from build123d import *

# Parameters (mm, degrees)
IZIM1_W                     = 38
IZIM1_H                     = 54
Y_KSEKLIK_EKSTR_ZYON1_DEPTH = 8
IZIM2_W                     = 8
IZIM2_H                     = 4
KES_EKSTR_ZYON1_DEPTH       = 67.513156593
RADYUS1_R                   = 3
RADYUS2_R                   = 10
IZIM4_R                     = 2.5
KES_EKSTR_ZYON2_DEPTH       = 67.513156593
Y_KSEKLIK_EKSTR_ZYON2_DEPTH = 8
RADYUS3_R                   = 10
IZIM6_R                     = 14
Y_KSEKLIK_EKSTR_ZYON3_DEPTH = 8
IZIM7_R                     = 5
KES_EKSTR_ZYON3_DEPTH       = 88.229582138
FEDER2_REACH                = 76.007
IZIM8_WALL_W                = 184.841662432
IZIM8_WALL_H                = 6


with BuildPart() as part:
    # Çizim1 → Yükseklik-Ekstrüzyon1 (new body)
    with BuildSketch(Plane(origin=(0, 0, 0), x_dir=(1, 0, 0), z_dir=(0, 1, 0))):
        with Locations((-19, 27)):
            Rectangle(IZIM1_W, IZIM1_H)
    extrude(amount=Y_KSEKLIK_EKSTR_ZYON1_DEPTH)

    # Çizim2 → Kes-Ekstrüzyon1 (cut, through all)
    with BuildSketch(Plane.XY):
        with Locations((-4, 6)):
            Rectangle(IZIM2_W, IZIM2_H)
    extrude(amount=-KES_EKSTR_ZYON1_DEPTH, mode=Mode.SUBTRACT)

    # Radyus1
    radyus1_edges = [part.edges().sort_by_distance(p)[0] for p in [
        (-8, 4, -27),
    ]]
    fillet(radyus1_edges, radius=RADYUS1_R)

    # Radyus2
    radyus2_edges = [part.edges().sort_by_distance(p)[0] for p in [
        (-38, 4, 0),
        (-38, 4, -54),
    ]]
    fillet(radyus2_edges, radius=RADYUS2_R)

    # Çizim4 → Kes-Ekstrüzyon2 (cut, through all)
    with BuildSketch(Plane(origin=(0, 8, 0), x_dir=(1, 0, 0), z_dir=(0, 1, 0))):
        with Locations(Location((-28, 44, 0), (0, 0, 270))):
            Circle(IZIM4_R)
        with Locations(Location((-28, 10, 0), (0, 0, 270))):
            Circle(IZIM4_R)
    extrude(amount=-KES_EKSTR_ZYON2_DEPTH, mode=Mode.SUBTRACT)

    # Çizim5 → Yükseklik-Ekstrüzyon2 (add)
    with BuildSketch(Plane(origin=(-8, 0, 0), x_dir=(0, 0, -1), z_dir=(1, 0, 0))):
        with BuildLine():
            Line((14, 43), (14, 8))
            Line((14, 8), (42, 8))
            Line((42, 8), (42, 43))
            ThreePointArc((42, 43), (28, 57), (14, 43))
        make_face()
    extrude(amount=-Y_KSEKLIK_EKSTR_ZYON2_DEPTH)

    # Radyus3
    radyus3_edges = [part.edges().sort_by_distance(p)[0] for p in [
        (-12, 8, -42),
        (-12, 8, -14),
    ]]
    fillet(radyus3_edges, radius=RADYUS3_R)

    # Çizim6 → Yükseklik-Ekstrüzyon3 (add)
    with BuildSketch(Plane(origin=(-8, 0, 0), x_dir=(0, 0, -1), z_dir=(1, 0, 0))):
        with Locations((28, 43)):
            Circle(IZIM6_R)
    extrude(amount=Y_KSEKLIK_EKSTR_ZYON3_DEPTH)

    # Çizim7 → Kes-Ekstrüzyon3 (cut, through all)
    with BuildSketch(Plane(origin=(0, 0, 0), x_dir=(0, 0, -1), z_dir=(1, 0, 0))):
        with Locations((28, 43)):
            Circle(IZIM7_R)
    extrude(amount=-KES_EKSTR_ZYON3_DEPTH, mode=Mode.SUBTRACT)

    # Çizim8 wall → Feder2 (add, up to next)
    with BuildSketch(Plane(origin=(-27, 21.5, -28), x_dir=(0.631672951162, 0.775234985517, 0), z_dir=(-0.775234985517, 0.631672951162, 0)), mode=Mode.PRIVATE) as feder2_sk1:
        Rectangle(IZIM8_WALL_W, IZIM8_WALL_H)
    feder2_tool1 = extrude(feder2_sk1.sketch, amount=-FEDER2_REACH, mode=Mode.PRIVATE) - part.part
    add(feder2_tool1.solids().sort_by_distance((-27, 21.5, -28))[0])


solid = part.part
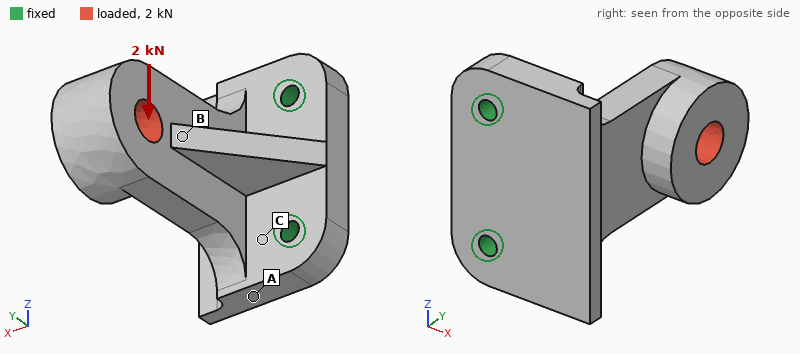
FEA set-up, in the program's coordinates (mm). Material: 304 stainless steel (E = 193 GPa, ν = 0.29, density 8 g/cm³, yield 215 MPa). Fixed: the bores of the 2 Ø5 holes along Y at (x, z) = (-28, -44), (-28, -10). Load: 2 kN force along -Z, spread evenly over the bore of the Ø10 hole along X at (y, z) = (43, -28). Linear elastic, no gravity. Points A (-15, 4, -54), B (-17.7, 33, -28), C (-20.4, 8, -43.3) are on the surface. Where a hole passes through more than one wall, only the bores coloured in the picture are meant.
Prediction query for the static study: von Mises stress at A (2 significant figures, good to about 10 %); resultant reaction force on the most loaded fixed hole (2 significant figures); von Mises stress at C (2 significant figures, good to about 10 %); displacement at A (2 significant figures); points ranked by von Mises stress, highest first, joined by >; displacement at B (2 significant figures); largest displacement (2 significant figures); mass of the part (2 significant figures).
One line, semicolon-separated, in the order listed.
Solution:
25 MPa; 2.7 kN; 37 MPa; 9.7 µm; C > A > B; 23 µm; 51 µm; 240 g
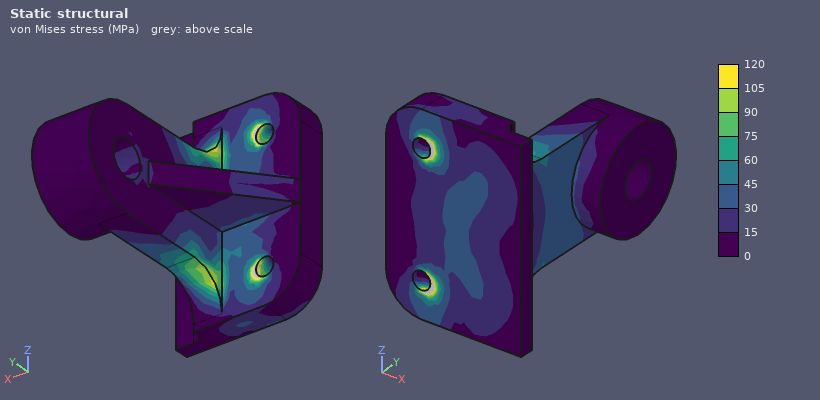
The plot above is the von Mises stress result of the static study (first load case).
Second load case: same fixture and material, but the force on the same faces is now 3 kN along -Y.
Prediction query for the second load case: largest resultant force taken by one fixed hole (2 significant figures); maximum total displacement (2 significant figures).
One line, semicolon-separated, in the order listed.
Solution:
1.6 kN; 84 µm
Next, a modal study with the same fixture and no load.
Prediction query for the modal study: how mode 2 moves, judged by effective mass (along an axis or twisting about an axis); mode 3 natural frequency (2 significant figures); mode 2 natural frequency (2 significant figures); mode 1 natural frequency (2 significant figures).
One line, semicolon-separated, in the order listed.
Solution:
along Z; 7900 Hz; 4000 Hz; 2300 Hz
